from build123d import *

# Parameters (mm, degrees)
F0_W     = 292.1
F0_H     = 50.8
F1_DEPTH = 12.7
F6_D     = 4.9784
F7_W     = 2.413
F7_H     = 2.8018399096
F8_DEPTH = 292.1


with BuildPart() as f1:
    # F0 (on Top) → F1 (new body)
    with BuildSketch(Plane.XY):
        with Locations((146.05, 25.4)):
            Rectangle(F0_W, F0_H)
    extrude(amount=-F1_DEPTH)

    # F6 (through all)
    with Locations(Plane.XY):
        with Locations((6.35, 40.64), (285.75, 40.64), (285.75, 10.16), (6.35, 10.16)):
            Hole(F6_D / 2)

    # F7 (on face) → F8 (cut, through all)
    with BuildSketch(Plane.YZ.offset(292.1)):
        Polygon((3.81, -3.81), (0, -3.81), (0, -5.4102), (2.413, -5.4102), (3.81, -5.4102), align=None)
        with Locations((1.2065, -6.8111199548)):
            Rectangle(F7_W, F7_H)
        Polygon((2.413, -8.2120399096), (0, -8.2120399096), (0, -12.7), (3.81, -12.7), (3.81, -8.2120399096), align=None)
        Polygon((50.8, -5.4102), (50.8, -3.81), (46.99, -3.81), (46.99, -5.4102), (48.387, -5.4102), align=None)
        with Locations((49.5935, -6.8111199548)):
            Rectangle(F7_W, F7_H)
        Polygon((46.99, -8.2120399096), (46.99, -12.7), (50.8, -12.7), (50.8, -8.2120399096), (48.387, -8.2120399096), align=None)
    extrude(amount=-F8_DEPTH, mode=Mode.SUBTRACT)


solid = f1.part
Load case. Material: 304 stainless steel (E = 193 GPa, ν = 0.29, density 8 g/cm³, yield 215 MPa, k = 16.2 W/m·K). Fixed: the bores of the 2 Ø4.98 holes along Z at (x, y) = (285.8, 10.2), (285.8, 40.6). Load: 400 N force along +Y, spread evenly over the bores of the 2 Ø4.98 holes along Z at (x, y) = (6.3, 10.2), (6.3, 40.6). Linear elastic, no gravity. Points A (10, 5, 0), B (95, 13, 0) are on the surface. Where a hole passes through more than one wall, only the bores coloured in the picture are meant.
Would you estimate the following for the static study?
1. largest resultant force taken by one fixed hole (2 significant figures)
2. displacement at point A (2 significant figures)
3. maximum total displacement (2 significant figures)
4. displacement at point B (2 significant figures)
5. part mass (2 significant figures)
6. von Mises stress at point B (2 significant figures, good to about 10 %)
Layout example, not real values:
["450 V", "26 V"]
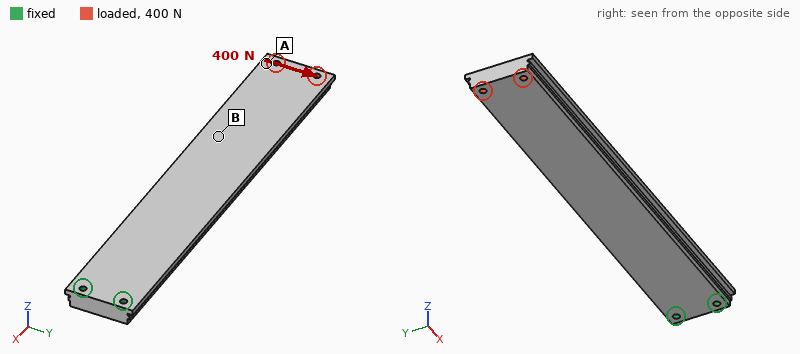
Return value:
["3.4 kN", "0.15 mm", "0.16 mm", "0.082 mm", "1.4 kg", "4.5 MPa"]
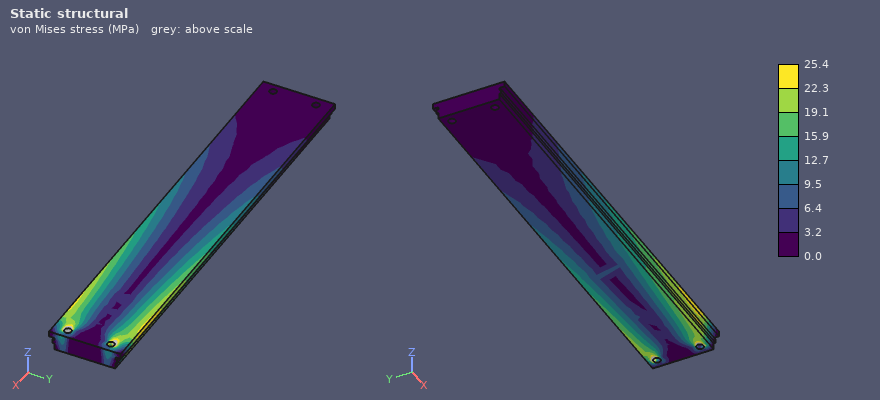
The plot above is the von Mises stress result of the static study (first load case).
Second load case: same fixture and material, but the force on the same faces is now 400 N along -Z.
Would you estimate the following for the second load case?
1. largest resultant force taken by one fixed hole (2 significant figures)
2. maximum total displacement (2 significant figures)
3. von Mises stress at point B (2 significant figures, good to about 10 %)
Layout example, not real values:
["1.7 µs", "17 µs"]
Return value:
["340 N", "2.0 mm", "28 MPa"]
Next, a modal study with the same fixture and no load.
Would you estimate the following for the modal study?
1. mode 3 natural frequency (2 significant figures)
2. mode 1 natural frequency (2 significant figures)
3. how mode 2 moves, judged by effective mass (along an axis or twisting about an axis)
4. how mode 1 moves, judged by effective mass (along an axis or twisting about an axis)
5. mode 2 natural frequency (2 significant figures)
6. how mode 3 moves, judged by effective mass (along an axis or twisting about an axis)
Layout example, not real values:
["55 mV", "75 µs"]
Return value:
["760 Hz", "120 Hz", "along Y", "along Z", "440 Hz", "along Z"]
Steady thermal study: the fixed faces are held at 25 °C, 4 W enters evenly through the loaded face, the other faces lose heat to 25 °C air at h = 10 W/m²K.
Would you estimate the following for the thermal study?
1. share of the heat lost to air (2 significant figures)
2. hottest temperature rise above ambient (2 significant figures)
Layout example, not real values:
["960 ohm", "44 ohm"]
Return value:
["94 %", "34 K"]
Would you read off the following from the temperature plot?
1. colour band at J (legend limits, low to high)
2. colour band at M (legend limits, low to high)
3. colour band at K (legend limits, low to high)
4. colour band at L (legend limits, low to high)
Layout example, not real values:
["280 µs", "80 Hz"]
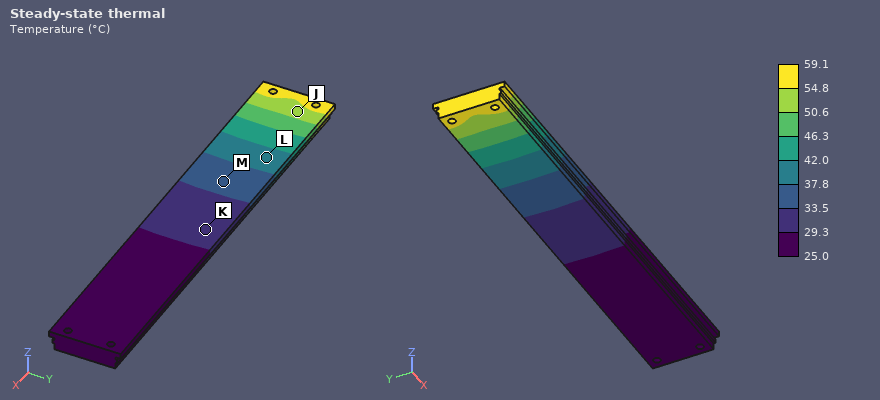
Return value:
["50.6 to 54.8 °C", "33.5 to 37.8 °C", "29.3 to 33.5 °C", "37.8 to 42.0 °C"]
